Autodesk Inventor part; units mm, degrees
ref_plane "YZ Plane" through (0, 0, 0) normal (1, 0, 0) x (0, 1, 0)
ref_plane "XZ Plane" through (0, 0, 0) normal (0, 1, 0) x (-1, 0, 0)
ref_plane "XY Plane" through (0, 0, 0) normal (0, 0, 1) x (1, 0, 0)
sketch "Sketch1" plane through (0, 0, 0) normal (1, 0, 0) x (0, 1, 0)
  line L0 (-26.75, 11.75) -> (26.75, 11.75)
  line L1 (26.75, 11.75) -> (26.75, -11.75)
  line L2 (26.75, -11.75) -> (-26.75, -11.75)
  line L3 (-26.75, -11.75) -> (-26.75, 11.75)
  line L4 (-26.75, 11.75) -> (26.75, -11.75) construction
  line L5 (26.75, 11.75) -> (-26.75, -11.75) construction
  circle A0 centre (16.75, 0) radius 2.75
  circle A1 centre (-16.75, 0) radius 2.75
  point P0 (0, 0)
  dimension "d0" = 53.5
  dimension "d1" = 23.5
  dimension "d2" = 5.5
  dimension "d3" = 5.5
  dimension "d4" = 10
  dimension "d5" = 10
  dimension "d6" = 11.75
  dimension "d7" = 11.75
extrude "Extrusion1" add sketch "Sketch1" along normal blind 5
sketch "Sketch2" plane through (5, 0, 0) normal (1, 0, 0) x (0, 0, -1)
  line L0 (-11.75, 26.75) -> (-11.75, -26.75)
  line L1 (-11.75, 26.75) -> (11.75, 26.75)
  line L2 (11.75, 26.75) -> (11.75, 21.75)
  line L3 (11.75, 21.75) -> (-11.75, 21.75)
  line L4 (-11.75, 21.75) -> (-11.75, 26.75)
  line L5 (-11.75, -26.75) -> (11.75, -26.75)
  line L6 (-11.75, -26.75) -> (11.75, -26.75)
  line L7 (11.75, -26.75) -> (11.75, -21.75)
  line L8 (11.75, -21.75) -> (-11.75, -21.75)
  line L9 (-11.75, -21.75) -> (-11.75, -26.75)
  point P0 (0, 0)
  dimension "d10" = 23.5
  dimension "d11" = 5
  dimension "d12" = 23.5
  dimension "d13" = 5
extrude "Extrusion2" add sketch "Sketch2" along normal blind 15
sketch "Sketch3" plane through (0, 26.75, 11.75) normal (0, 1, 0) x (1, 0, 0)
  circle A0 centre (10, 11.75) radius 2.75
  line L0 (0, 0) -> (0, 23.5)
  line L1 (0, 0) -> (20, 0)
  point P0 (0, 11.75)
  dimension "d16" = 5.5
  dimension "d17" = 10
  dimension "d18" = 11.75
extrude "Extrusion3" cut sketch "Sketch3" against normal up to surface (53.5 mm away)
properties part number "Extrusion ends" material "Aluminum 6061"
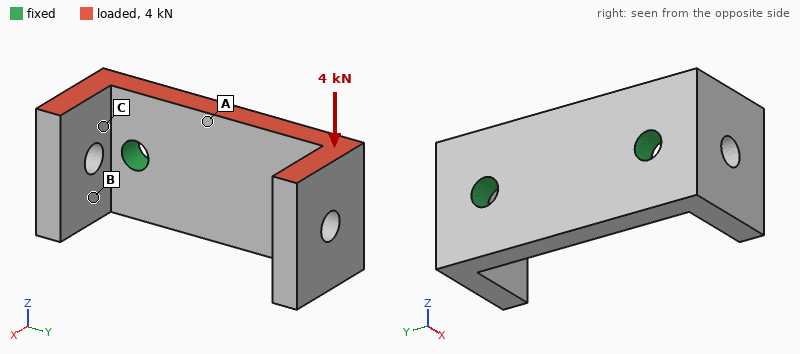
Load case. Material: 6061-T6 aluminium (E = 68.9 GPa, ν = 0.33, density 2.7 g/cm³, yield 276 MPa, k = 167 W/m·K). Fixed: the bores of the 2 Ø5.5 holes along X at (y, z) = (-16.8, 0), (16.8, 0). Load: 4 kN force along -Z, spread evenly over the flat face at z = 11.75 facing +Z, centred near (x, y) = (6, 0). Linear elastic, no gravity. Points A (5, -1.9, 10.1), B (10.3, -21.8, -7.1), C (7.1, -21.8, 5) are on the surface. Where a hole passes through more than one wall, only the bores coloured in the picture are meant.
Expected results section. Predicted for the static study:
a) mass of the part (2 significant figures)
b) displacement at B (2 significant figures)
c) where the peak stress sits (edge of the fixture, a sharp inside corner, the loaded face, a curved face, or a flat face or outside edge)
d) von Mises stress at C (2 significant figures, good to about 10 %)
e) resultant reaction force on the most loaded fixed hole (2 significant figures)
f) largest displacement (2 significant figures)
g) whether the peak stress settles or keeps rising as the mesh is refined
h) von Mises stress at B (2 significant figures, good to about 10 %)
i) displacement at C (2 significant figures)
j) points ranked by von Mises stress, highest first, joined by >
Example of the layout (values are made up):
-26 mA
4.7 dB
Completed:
25 g
20 µm
edge of the fixture
34 MPa
2.0 kN
42 µm
keeps rising
20 MPa
13 µm
C > B > A
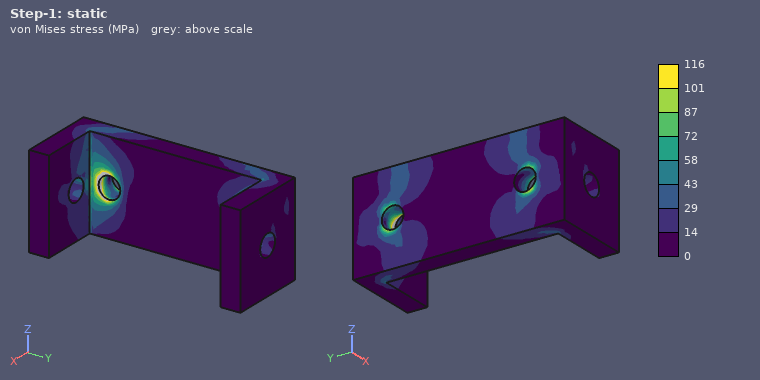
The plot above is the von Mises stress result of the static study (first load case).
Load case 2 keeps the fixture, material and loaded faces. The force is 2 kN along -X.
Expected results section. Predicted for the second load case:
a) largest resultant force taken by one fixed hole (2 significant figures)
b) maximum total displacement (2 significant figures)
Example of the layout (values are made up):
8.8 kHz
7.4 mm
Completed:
1.0 kN
45 µm
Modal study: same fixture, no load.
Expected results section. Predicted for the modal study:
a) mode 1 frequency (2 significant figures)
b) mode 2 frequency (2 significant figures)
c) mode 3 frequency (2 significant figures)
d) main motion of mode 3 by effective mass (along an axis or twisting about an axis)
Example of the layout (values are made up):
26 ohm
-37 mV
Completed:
8300 Hz
8300 Hz
11 kHz
along Z
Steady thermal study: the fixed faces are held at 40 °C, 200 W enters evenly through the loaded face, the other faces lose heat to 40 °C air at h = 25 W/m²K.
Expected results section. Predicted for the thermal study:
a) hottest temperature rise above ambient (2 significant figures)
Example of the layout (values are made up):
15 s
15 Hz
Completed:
67 K
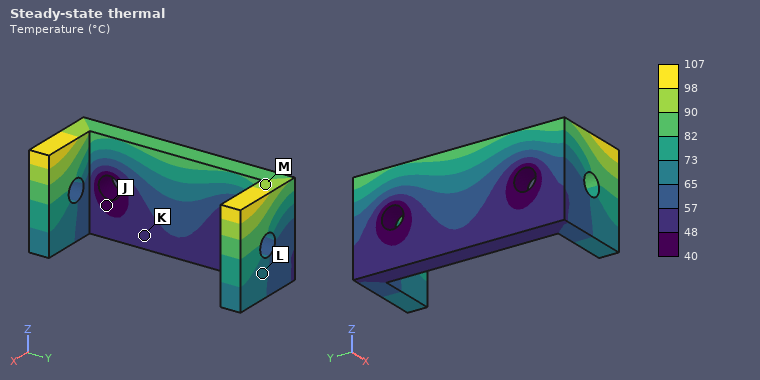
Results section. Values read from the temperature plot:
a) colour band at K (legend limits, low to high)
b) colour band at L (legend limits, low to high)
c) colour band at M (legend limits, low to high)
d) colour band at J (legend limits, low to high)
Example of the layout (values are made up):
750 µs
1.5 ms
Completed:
48 to 57 °C
65 to 73 °C
90 to 98 °C
40 to 48 °C
